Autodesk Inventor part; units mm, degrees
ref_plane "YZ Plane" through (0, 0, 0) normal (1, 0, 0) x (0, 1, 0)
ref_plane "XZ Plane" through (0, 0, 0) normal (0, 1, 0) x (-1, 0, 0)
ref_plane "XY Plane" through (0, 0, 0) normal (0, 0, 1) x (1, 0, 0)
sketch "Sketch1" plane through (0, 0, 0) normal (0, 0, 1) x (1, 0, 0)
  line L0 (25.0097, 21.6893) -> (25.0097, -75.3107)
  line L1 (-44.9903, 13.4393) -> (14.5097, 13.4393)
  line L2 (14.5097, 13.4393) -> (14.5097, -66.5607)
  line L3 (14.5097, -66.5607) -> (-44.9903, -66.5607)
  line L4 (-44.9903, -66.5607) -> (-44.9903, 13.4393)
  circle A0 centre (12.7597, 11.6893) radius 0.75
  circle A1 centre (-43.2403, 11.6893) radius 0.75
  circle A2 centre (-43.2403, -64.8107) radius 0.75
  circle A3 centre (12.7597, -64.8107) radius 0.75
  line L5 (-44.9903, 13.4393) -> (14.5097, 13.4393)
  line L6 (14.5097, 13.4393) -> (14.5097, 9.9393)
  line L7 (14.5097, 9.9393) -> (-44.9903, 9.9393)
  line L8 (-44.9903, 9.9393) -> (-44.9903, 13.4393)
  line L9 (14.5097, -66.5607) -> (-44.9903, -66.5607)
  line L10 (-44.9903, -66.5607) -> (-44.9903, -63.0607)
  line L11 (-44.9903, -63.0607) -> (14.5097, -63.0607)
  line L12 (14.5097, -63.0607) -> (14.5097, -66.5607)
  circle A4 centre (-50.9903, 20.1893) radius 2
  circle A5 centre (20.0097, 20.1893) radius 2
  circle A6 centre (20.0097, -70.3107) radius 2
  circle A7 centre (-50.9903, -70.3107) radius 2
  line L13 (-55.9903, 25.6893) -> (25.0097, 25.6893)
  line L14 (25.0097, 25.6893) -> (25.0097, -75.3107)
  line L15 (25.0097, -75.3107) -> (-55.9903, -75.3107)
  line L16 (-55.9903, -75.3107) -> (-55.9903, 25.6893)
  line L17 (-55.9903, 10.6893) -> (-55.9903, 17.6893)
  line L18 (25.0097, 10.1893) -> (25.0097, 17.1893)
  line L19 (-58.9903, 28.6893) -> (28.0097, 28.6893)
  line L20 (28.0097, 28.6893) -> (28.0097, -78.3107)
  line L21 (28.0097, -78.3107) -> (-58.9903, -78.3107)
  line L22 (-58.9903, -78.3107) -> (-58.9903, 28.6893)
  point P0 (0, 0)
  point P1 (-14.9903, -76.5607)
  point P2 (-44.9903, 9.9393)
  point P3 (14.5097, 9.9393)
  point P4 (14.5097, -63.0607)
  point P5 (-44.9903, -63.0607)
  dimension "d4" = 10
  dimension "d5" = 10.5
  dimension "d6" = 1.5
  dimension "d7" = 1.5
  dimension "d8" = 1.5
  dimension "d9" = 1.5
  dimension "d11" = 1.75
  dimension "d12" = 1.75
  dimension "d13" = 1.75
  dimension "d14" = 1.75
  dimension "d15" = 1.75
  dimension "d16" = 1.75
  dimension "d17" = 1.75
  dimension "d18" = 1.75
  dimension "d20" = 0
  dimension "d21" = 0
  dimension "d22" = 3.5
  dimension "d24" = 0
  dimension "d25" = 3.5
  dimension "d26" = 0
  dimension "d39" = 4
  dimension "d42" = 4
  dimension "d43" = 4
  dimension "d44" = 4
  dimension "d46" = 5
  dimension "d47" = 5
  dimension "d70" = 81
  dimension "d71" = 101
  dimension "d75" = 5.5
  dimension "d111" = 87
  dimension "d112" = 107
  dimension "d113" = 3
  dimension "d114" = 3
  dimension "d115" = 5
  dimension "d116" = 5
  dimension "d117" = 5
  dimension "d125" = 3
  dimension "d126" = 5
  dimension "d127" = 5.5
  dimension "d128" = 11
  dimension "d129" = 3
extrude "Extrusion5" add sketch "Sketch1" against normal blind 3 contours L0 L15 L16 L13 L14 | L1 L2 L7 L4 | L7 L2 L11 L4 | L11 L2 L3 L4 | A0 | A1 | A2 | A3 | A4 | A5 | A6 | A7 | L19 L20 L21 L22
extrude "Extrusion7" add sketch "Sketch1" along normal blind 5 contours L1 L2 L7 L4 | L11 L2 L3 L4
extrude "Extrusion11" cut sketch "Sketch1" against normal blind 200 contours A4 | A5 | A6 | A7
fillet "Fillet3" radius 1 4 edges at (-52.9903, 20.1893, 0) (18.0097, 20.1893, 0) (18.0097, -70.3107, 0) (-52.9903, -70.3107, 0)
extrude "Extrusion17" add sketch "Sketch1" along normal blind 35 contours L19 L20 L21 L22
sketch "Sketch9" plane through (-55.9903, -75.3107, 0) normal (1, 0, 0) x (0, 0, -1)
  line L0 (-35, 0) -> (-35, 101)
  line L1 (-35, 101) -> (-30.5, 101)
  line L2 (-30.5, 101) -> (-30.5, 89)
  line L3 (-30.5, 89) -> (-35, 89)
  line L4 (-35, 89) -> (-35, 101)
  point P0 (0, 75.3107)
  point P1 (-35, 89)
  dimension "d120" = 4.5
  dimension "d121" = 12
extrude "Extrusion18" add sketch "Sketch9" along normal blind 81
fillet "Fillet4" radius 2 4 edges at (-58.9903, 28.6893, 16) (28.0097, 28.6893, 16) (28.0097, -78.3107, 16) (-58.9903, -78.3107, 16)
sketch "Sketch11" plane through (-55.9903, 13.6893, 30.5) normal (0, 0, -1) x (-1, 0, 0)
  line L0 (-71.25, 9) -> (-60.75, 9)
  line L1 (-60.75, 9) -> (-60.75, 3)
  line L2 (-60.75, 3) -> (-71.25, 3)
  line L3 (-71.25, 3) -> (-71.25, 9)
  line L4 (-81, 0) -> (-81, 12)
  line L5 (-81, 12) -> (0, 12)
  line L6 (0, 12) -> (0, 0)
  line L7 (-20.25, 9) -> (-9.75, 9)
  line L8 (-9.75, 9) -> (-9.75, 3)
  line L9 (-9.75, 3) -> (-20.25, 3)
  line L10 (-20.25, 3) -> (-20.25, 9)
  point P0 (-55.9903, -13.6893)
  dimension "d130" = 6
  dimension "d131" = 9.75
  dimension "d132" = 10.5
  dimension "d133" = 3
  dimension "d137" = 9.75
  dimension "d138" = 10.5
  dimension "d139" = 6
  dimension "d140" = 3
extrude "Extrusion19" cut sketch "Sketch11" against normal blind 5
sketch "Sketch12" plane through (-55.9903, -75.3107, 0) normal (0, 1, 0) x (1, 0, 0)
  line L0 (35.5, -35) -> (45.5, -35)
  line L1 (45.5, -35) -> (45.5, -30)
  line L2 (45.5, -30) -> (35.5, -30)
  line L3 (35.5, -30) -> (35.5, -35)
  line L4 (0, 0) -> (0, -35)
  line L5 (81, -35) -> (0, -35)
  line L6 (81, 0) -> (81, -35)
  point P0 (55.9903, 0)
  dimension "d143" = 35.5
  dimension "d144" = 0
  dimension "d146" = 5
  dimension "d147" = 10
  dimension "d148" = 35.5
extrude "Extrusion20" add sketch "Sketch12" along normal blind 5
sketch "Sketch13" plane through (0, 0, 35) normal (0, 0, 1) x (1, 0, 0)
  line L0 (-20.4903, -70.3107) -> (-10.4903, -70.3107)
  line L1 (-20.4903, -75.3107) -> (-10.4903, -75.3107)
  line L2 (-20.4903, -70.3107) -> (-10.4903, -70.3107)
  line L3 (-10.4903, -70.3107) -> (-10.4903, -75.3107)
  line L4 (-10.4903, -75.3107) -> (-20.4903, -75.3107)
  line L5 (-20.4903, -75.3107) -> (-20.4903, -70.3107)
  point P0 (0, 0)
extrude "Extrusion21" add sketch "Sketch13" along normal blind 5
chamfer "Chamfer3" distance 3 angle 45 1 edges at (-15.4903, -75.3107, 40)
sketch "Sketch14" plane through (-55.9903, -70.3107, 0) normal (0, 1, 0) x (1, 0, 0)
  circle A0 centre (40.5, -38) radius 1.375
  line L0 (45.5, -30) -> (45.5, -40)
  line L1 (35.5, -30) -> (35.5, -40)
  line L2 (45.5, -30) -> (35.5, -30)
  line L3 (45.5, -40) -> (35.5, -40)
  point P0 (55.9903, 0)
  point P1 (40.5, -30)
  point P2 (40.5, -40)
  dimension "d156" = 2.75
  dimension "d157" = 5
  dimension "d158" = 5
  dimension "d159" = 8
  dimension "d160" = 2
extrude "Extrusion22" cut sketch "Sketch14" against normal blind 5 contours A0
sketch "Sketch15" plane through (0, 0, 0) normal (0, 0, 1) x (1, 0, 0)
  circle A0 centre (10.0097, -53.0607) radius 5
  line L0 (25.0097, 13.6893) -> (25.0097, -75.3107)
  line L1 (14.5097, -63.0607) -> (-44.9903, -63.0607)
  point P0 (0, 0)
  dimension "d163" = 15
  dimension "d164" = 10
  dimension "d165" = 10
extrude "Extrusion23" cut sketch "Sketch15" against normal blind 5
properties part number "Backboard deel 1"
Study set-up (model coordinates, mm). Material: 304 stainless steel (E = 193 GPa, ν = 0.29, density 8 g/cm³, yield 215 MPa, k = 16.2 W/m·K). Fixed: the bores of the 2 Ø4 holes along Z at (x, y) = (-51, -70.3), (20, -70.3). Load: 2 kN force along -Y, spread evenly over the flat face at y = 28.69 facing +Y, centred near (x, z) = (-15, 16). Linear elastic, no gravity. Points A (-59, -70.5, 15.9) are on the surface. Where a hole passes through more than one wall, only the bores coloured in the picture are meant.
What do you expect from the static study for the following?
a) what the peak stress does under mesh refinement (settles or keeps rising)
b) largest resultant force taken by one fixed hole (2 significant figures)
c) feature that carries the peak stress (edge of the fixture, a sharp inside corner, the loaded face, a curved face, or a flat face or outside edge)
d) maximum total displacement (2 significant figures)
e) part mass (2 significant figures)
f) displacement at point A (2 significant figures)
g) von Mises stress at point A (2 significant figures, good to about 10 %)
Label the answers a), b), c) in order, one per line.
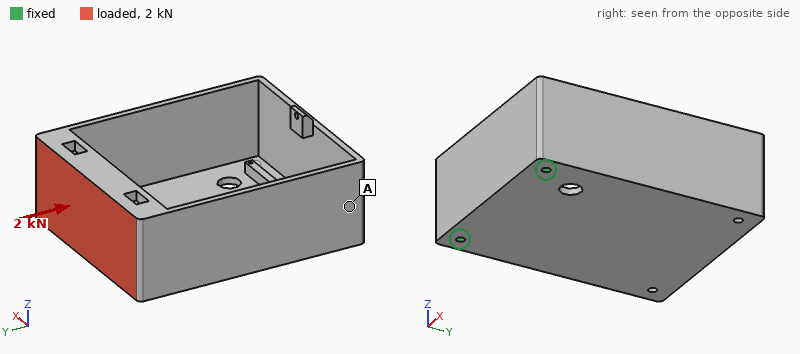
a) keeps rising
b) 1.0 kN
c) edge of the fixture
d) 0.60 mm
e) 590 g
f) 0.097 mm
g) 25 MPa
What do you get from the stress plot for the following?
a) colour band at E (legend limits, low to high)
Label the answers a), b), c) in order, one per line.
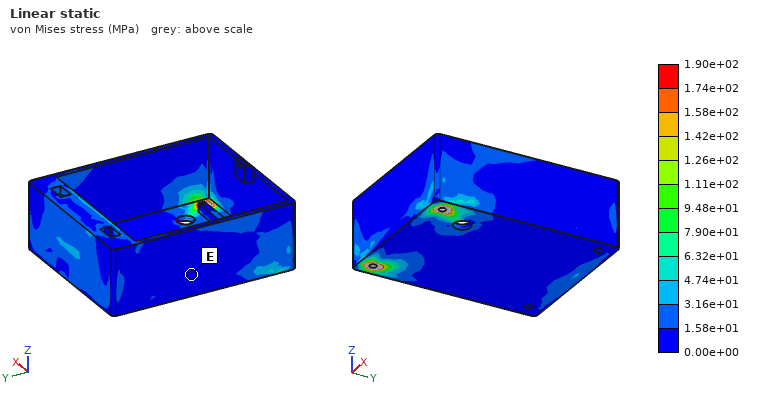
a) 0.00e+00 to 1.58e+01 MPa
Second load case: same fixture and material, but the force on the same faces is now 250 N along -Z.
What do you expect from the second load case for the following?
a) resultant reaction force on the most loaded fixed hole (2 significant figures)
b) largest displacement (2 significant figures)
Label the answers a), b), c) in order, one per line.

a) 130 N
b) 0.42 mm
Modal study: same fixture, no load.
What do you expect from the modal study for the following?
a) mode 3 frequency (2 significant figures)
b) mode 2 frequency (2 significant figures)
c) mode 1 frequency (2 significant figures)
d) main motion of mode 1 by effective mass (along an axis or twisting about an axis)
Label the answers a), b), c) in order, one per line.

a) 2100 Hz
b) 560 Hz
c) 260 Hz
d) along Z
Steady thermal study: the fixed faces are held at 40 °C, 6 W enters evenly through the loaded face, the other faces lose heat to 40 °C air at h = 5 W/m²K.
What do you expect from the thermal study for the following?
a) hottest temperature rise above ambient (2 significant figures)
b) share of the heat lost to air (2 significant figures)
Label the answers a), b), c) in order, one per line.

a) 49 K
b) 75 %
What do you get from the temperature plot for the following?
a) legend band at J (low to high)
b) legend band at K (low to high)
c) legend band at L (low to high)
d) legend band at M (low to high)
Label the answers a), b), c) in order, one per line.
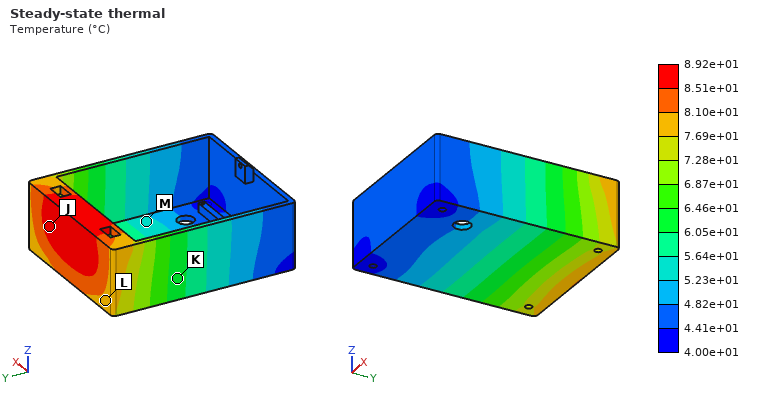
a) 8.51e+01 to 8.92e+01 °C
b) 6.05e+01 to 6.46e+01 °C
c) 7.69e+01 to 8.10e+01 °C
d) 5.23e+01 to 5.64e+01 °C
